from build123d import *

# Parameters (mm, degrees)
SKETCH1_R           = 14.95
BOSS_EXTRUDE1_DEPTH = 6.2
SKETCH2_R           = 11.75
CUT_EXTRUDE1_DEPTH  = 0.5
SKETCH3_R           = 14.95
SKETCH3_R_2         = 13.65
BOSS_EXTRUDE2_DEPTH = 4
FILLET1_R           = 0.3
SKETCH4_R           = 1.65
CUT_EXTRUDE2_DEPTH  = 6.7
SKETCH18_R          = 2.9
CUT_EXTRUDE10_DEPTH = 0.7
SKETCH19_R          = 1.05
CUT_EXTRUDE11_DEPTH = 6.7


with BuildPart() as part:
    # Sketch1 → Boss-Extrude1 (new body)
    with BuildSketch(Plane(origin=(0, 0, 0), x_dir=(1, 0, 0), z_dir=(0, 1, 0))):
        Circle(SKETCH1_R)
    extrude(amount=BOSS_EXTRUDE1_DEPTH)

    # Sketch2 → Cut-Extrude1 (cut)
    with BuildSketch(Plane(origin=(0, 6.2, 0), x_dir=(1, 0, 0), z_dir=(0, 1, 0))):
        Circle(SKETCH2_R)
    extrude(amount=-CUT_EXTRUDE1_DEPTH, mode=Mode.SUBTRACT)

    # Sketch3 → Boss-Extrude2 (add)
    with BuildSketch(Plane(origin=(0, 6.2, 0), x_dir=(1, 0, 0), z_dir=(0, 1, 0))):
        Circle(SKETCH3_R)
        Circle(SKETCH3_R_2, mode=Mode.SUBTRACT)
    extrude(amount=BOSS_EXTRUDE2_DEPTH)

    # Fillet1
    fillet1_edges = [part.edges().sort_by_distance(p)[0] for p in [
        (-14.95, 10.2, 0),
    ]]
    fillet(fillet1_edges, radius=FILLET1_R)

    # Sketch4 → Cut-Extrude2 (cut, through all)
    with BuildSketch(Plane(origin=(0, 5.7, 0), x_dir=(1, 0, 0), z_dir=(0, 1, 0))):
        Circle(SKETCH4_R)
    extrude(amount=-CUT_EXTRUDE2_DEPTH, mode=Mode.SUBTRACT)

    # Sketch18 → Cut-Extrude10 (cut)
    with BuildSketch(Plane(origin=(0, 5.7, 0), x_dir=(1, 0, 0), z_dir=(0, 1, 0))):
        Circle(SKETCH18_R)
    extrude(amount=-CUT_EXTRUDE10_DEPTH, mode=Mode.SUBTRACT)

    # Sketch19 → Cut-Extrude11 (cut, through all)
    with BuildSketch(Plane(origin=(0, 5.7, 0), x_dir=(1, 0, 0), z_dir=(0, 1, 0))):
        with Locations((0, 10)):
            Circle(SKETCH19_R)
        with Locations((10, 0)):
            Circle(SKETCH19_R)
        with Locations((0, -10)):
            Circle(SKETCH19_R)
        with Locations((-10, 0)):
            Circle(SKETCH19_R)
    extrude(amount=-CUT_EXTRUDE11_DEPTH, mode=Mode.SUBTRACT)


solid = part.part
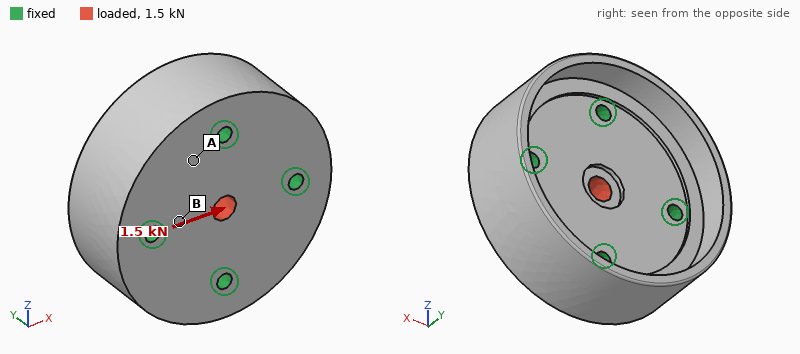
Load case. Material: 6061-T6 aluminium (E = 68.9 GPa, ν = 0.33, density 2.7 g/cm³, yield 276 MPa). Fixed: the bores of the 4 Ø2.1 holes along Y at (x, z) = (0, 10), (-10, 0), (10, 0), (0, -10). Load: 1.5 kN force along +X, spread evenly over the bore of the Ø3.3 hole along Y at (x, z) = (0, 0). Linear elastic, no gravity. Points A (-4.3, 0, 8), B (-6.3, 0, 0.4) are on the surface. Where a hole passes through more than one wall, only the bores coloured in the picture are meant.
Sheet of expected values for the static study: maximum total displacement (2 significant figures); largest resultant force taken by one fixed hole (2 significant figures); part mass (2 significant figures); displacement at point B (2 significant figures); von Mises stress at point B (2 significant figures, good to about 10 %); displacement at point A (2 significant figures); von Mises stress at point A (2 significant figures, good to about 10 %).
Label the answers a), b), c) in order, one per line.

a) 2.4 µm
b) 500 N
c) 12 g
d) 0.80 µm
e) 19 MPa
f) 0.51 µm
g) 4.2 MPa
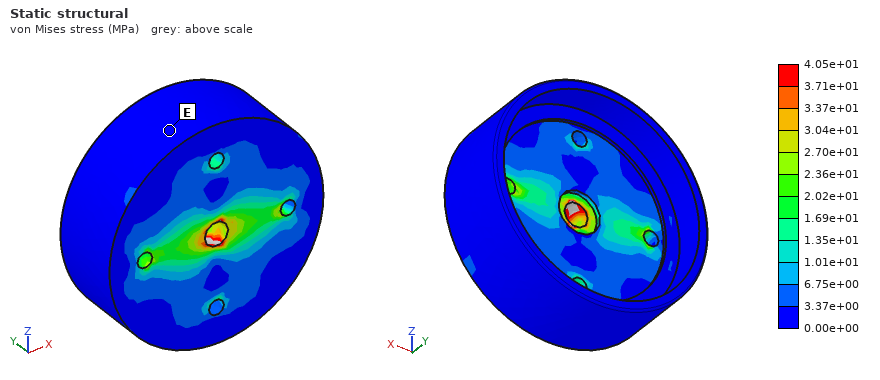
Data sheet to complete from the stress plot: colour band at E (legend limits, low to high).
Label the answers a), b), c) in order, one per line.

a) 0.00e+00 to 3.37e+00 MPa
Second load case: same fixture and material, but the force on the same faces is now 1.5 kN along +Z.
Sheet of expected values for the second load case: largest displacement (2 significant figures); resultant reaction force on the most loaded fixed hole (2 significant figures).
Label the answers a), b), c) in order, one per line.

a) 2.4 µm
b) 500 N
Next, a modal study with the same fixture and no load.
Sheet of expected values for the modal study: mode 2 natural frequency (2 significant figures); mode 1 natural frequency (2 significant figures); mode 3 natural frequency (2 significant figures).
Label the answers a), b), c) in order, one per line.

a) 44 kHz
b) 39 kHz
c) 44 kHz
